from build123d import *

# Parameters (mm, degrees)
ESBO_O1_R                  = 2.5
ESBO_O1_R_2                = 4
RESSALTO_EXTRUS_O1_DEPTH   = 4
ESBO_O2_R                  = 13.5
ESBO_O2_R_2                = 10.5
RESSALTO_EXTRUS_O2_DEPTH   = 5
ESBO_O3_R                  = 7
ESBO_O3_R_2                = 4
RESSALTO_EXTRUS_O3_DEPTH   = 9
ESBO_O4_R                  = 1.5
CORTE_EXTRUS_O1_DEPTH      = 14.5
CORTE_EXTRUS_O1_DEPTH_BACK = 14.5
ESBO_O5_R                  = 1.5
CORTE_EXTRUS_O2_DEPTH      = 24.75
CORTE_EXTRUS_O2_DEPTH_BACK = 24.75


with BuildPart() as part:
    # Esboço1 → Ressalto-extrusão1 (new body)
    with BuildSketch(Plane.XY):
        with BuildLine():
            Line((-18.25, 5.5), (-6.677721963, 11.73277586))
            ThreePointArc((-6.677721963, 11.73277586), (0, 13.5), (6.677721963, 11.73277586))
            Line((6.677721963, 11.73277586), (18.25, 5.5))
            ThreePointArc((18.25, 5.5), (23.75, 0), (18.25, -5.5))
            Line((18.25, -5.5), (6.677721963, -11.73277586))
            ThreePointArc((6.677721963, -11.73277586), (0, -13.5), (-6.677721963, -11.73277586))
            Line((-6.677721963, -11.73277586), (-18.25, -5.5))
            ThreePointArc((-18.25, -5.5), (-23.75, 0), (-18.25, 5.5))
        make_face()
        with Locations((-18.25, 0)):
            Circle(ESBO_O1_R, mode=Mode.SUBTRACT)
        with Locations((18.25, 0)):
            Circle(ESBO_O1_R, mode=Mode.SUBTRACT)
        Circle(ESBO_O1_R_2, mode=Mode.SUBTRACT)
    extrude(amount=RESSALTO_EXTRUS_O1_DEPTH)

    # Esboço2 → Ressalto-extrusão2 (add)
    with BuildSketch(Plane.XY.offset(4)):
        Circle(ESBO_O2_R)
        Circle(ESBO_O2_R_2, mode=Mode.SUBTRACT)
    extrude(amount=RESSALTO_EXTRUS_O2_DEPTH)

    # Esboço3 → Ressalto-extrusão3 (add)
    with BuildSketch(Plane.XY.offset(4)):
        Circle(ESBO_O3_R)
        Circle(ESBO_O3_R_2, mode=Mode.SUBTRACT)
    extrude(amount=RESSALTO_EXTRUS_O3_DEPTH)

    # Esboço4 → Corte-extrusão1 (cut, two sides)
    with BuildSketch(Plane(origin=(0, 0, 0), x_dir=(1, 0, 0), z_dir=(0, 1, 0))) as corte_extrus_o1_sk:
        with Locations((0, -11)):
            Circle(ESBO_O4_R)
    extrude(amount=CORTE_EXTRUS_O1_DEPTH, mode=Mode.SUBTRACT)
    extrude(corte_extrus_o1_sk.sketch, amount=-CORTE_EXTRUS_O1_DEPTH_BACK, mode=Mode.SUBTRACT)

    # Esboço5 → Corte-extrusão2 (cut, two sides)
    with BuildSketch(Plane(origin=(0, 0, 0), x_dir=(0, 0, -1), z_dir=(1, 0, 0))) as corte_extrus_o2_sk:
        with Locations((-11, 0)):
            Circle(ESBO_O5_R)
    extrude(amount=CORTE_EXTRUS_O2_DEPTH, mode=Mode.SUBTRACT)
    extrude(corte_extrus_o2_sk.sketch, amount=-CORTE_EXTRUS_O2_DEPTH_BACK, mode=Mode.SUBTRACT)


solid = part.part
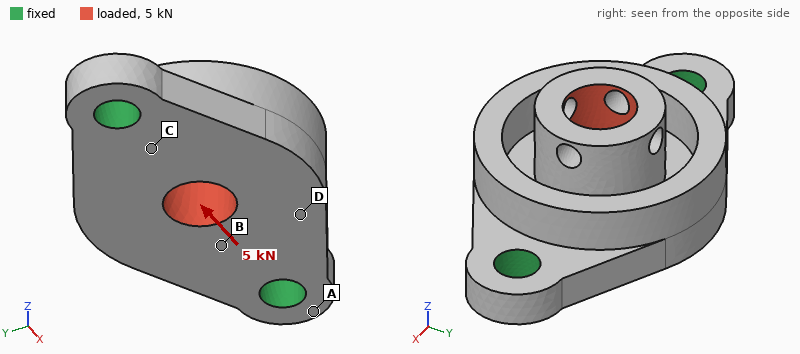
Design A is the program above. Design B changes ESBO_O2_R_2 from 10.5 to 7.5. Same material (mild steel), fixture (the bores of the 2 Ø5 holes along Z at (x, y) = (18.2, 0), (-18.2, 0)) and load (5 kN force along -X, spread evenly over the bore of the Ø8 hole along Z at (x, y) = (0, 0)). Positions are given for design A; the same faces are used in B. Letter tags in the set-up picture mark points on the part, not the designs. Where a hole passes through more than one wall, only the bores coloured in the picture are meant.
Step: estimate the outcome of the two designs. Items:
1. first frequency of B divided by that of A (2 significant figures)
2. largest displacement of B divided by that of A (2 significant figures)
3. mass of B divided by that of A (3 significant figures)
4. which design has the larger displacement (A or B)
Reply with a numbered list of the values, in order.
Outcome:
1. 0.98
2. 0.81
3. 1.17
4. A
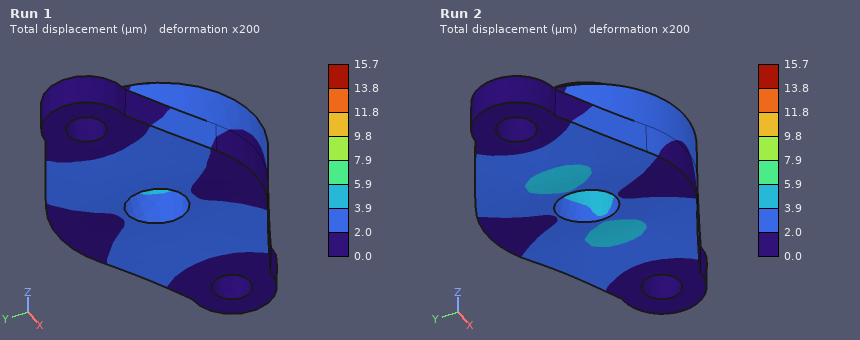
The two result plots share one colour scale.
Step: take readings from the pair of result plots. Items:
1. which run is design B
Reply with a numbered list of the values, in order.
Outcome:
1. Run 1
